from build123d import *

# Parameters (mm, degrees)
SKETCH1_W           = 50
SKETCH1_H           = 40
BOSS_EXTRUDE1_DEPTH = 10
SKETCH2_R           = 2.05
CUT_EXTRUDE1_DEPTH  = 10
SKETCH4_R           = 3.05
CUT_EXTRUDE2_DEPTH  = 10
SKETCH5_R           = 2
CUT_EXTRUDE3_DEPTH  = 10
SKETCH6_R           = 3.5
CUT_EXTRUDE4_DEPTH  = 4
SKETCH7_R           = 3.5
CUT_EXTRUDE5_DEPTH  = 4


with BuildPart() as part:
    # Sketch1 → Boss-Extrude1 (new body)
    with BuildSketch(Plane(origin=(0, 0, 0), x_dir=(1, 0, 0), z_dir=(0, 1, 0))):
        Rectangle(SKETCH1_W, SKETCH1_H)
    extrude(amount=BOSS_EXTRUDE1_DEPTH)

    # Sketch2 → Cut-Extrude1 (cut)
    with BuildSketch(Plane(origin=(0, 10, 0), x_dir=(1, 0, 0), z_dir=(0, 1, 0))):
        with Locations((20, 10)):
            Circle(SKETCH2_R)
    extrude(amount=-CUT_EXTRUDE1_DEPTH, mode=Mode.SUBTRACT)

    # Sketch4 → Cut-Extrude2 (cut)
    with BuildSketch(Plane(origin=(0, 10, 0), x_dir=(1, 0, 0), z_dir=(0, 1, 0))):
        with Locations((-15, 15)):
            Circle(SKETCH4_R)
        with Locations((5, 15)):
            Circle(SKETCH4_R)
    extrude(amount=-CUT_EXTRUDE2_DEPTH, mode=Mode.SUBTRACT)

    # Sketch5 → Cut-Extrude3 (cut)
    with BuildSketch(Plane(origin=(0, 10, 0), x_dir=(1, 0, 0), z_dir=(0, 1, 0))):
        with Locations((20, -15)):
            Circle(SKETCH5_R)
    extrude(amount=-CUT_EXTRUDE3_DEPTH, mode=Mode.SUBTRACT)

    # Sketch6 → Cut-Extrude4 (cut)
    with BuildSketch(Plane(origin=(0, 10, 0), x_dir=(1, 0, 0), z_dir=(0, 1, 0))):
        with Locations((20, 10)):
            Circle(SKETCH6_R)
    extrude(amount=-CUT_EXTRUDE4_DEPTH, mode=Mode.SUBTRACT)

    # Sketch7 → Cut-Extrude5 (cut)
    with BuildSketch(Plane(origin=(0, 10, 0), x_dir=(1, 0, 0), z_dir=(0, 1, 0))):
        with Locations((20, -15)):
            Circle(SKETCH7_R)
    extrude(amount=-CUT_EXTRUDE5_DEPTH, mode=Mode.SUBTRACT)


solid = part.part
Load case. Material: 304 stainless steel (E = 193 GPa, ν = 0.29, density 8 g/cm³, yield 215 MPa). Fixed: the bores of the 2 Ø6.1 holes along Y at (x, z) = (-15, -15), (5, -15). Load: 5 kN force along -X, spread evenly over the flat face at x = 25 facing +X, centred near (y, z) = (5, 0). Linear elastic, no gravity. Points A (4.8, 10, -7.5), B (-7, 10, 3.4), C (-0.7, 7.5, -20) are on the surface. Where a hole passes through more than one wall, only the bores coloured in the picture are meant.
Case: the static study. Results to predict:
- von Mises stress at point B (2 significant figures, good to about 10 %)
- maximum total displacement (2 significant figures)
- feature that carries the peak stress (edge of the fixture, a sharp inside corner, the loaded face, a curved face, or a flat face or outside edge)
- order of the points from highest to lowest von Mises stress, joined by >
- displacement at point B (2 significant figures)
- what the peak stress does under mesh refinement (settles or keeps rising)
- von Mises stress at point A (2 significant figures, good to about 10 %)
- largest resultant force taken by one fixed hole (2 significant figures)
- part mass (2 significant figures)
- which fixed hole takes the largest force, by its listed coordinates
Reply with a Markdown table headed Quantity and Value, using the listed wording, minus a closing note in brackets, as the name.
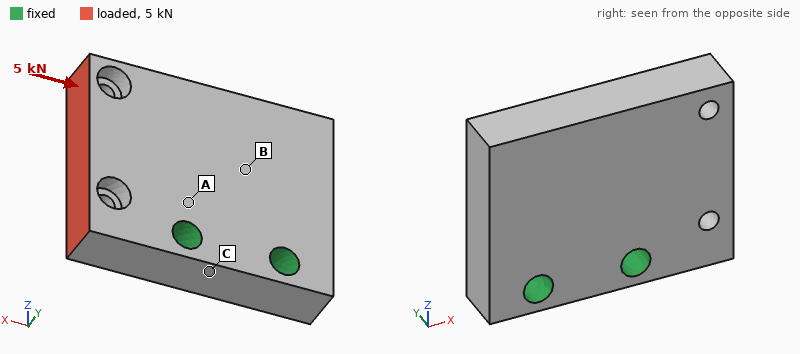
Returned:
| Quantity | Value |
|---|---|
| von Mises stress at point B | 16 MPa |
| maximum total displacement | 11 µm |
| feature that carries the peak stress | edge of the fixture |
| order of the points from highest to lowest von Mises stress, joined by > | A > B > C |
| displacement at point B | 3.5 µm |
| what the peak stress does under mesh refinement | keeps rising |
| von Mises stress at point A | 30 MPa |
| largest resultant force taken by one fixed hole | 4.3 kN |
| part mass | 150 g |
| which fixed hole takes the largest force, by its listed coordinates | (5, -15) |
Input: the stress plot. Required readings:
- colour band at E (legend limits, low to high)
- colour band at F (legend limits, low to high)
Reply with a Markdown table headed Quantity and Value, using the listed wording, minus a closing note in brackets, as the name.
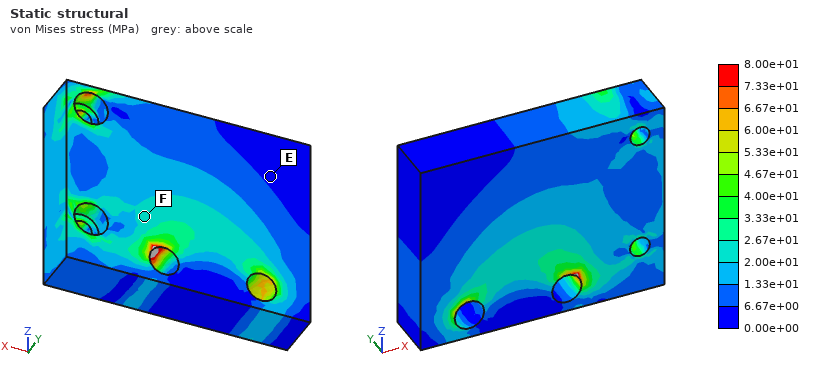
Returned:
| Quantity | Value |
|---|---|
| colour band at E | 0.00e+00 to 6.67e+00 MPa |
| colour band at F | 2.00e+01 to 2.67e+01 MPa |
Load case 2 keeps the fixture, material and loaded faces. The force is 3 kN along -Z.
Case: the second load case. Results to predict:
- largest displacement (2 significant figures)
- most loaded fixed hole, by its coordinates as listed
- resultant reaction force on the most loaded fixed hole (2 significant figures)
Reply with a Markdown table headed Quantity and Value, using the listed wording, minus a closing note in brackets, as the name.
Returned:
| Quantity | Value |
|---|---|
| largest displacement | 12 µm |
| most loaded fixed hole, by its coordinates as listed | (5, -15) |
| resultant reaction force on the most loaded fixed hole | 5.0 kN |
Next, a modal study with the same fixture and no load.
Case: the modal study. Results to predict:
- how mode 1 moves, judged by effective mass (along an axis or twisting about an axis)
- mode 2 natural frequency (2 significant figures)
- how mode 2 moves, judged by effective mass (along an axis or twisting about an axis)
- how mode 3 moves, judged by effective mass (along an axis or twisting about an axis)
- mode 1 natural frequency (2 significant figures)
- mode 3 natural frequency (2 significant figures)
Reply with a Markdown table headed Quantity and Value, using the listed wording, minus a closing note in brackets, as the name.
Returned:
| Quantity | Value |
|---|---|
| how mode 1 moves, judged by effective mass | along Y |
| mode 2 natural frequency | 9500 Hz |
| how mode 2 moves, judged by effective mass | twisting about Z |
| how mode 3 moves, judged by effective mass | along X |
| mode 1 natural frequency | 5800 Hz |
| mode 3 natural frequency | 12 kHz |
